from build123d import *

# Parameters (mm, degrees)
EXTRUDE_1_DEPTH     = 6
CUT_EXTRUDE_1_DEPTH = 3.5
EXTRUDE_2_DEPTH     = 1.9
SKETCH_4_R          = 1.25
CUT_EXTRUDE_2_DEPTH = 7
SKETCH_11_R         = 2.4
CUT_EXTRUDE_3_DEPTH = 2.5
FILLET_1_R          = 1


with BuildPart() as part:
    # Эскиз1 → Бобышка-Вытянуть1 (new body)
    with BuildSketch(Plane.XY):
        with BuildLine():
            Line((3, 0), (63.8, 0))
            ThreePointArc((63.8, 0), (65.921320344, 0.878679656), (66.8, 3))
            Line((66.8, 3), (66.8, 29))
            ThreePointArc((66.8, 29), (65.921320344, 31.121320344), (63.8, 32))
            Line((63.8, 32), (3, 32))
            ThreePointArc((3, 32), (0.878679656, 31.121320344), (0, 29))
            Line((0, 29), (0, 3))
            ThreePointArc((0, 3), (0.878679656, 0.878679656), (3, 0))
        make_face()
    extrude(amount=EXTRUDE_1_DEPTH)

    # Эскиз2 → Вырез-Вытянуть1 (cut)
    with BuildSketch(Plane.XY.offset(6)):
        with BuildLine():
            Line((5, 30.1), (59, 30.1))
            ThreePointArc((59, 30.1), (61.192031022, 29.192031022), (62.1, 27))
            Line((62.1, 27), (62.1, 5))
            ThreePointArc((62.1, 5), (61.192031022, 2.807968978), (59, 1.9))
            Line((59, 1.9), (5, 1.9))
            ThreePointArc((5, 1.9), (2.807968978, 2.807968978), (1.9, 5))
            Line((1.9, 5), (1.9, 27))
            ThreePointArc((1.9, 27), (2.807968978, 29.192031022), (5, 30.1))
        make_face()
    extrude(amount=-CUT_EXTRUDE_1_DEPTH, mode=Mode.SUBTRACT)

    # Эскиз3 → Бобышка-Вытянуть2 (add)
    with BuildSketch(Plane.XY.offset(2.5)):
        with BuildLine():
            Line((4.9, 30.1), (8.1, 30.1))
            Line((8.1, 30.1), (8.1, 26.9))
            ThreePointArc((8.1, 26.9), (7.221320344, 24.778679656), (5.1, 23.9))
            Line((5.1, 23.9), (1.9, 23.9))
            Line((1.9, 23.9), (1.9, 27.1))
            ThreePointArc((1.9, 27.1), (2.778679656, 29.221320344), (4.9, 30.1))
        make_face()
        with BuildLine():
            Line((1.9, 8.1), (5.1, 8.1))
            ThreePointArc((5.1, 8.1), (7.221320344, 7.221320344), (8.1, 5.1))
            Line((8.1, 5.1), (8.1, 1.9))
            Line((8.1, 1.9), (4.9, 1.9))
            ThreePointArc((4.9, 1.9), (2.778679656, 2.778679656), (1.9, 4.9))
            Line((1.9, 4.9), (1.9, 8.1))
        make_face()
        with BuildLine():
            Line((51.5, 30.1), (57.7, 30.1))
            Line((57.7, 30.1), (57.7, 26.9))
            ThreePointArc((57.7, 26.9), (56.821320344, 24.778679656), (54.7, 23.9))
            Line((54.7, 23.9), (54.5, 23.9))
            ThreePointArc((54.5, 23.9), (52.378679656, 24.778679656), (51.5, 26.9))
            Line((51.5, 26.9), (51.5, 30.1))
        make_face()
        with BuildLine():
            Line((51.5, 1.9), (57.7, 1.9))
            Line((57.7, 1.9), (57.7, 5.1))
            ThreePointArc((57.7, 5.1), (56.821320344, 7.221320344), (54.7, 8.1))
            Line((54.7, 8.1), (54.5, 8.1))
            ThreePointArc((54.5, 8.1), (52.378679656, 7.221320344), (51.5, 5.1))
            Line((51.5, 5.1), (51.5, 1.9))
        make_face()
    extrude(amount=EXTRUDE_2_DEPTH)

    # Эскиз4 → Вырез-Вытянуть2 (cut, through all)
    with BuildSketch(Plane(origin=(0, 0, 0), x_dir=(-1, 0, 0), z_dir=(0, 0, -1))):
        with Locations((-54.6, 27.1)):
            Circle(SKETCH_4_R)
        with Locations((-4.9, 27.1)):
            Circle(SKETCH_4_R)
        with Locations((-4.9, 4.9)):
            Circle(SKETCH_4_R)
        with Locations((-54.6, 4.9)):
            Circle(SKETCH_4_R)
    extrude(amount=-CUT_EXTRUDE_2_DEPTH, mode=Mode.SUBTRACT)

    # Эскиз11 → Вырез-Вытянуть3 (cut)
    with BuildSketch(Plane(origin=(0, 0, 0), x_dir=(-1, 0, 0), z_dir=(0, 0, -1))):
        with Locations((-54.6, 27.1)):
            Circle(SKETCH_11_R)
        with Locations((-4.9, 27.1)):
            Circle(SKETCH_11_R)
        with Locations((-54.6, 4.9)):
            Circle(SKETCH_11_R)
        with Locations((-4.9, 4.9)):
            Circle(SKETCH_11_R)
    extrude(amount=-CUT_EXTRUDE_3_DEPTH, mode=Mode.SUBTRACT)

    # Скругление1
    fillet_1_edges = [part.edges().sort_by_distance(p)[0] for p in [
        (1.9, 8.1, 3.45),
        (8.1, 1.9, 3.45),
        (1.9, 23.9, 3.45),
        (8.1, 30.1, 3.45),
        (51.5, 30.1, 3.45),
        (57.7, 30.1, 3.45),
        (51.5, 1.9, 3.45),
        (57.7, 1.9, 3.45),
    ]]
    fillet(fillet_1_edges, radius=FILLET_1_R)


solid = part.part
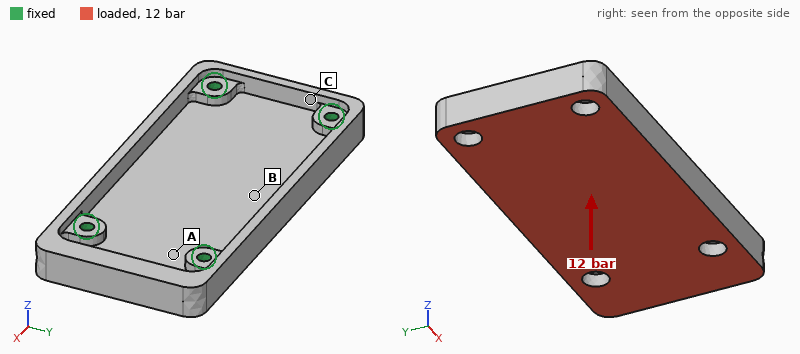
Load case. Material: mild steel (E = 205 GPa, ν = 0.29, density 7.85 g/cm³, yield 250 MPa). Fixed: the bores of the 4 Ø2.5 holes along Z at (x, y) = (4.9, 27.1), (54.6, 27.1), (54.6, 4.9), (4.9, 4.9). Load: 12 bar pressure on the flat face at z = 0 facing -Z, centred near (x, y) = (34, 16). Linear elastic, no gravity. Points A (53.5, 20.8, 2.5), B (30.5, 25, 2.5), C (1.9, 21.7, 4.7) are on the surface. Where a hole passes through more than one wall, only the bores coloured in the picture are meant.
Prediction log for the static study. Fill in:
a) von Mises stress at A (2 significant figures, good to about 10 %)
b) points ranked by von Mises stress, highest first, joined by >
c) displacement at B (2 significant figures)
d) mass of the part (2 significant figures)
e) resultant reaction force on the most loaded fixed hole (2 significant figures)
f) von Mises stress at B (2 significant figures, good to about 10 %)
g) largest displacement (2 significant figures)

62 MPa
A > B > C
40 µm
54 g
900 N
36 MPa
46 µm
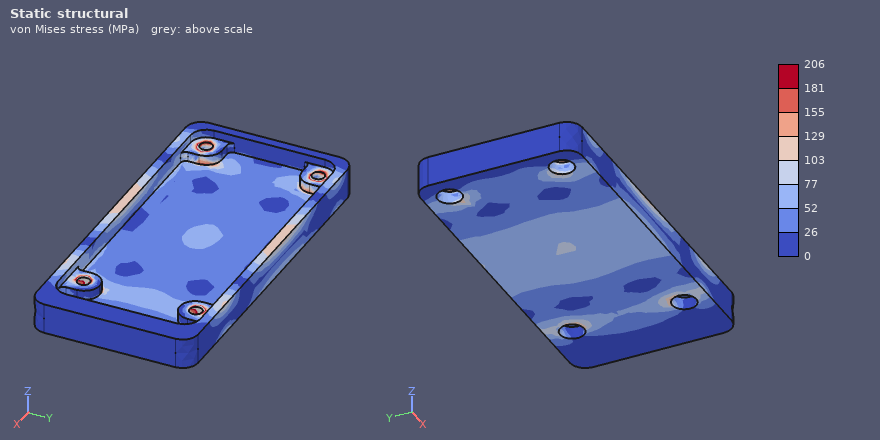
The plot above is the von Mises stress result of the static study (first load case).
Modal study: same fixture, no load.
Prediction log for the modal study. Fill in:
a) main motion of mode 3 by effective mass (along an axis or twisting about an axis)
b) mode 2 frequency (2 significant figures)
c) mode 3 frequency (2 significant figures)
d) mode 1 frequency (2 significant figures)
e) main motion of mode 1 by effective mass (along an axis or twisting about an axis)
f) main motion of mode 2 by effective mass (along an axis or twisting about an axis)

along Z
8900 Hz
10 kHz
6200 Hz
along Z
twisting about X
